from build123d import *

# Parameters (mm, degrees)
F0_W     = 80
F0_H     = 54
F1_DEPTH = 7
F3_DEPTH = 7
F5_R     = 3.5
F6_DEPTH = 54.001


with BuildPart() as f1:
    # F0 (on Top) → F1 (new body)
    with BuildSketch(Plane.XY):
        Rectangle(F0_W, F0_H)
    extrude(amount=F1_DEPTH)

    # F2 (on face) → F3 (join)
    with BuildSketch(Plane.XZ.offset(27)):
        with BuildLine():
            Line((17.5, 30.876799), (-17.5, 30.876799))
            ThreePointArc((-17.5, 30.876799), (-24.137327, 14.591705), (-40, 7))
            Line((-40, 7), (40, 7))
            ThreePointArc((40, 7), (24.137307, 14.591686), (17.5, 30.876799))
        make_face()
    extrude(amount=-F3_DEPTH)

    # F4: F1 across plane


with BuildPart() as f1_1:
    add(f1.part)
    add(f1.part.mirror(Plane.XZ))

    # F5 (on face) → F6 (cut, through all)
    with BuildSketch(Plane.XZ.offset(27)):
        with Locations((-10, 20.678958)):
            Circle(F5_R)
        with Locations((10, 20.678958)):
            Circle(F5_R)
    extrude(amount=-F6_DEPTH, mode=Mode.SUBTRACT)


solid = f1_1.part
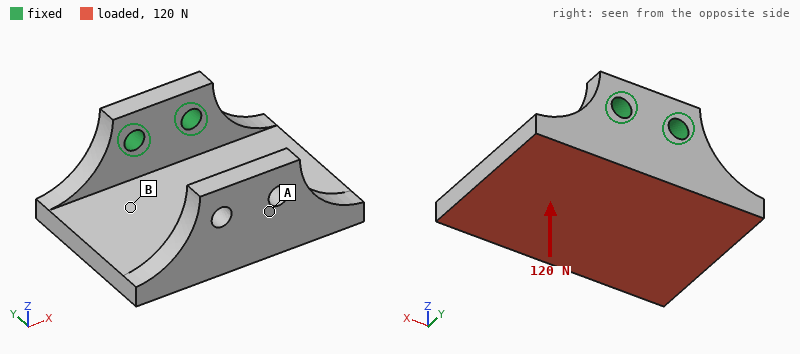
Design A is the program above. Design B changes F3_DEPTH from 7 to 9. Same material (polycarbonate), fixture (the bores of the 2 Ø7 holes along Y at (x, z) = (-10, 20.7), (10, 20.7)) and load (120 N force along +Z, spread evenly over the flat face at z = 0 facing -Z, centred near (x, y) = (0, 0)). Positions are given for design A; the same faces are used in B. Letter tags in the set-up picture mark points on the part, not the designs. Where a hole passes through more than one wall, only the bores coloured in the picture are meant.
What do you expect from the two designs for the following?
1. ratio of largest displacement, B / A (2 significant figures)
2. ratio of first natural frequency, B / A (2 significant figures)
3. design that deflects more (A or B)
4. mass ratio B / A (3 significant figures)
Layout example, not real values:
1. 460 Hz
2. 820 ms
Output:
1. 0.62
2. 1.2
3. A
4. 1.09
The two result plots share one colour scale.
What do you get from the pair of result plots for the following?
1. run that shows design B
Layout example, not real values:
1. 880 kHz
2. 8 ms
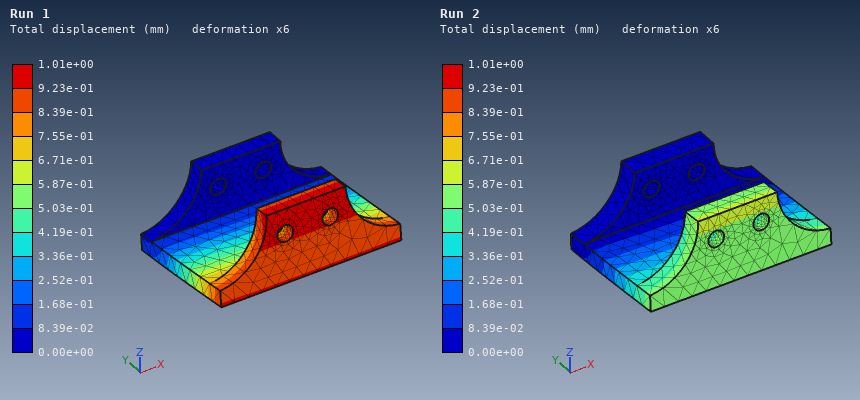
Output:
1. Run 2
